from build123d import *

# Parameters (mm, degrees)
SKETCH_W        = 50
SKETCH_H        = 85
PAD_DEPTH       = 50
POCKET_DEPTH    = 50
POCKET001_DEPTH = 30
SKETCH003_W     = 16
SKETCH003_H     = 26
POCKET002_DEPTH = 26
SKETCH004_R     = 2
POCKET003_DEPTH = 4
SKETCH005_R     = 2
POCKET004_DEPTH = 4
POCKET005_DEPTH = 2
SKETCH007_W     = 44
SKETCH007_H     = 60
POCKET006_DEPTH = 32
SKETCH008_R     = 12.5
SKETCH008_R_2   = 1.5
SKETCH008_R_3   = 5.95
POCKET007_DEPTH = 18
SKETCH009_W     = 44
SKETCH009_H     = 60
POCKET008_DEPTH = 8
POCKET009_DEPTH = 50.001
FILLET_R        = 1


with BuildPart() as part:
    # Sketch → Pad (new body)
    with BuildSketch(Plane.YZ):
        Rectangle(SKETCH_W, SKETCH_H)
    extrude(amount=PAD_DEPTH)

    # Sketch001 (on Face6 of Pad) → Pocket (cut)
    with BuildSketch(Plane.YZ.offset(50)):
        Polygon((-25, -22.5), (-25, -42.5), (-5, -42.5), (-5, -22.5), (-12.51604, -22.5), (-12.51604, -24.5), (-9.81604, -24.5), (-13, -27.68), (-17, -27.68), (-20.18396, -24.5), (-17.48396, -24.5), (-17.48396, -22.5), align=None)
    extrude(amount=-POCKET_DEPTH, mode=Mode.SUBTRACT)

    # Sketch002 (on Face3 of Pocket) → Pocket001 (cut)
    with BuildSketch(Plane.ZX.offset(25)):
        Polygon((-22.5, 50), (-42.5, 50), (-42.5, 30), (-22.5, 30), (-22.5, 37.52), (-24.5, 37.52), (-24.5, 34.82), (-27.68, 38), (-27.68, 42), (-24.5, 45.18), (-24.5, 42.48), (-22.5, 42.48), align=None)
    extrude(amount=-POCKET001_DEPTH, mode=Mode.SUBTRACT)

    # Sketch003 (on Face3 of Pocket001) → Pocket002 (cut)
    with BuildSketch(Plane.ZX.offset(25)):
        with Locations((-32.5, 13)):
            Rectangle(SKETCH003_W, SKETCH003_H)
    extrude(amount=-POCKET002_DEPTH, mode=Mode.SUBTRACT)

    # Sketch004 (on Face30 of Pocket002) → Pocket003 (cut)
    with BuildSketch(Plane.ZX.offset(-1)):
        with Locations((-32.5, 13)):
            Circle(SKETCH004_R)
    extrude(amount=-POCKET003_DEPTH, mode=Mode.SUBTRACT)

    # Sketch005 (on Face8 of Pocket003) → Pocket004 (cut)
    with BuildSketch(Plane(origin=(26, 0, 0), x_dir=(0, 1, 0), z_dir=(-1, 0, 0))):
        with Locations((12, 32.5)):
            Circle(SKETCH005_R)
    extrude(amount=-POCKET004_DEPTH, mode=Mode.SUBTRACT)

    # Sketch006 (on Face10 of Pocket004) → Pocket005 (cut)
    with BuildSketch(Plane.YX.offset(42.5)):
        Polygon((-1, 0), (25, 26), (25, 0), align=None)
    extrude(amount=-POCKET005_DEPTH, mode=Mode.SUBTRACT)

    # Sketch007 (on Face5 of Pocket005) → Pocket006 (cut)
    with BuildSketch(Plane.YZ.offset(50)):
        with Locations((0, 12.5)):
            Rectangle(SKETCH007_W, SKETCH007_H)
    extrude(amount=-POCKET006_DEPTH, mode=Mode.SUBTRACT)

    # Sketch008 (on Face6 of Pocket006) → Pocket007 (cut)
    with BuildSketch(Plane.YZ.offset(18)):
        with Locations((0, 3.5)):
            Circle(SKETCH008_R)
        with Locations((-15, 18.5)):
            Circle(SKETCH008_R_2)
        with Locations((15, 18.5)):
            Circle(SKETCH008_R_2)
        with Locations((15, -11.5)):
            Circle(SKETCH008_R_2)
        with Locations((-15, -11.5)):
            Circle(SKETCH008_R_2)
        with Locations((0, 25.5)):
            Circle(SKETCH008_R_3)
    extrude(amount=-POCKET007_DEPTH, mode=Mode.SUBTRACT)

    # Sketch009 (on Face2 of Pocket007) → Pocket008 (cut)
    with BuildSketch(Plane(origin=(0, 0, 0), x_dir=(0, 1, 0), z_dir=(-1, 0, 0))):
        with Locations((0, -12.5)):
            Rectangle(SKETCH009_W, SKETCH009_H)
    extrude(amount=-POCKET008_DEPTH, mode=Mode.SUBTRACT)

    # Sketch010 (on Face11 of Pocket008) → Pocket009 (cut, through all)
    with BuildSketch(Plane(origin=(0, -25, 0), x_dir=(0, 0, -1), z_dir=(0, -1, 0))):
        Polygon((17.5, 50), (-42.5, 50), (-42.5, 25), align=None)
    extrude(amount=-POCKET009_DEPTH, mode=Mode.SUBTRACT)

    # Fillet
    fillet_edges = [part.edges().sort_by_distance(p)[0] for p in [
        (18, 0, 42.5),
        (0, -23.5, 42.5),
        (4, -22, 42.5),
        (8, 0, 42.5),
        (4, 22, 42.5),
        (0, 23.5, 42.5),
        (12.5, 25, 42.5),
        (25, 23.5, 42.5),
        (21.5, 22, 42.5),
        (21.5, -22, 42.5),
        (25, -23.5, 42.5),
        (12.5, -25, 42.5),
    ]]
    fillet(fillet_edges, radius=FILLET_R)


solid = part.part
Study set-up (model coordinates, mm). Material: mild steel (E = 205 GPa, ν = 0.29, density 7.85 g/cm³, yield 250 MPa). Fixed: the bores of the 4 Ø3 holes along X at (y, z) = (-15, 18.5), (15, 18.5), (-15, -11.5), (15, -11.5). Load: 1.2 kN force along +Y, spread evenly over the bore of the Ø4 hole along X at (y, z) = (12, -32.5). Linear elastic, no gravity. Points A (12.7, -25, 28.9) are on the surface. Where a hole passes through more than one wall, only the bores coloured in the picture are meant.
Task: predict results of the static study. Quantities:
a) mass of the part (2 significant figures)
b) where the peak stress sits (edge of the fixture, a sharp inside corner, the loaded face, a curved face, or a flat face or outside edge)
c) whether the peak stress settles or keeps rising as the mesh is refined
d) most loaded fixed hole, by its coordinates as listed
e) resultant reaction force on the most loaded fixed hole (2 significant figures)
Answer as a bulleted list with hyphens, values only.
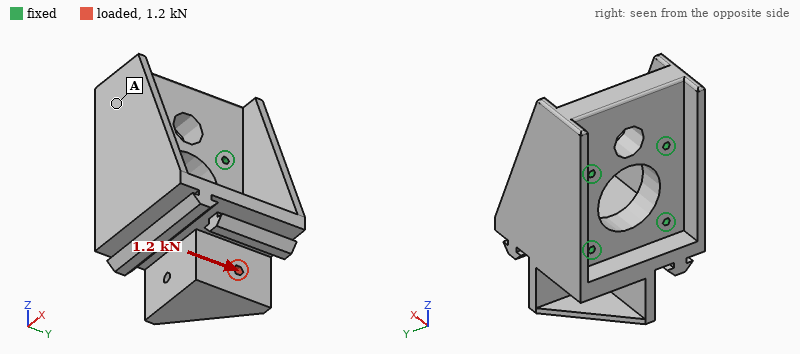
- 430 g
- a sharp inside corner
- keeps rising
- (-15, -11.5)
- 1.0 kN
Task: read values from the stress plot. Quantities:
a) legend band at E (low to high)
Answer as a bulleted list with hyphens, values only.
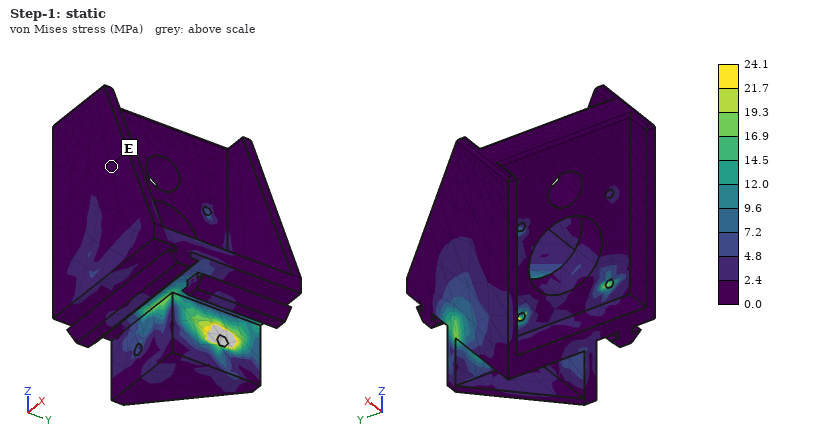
- 0.0 to 2.4 MPa
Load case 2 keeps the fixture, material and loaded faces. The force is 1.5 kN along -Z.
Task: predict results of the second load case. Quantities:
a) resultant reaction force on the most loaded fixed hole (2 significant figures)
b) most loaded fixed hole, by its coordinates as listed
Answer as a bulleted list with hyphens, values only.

- 960 N
- (15, -11.5)
